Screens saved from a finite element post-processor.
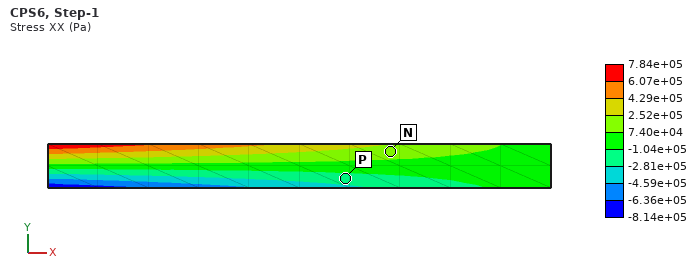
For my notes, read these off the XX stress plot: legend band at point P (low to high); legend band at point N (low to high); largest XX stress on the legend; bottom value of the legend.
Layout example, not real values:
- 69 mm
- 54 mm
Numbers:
- -2.81e+05 to -1.04e+05 Pa
- 7.40e+04 to 2.52e+05 Pa
- 7.84e+05 Pa
- -8.14e+05 Pa
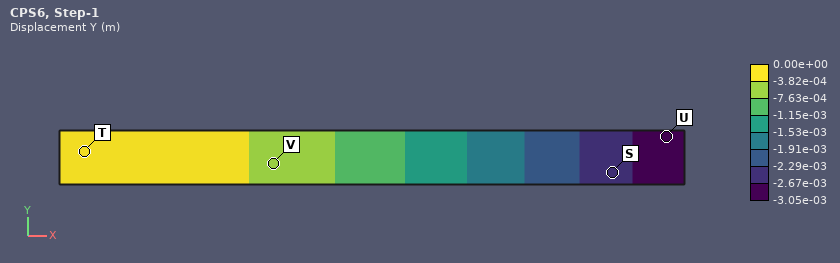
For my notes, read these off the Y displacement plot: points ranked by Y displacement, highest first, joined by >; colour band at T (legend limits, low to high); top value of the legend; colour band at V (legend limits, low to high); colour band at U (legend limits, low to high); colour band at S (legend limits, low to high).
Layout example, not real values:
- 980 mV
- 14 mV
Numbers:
- T > V > S > U
- -3.82e-04 to 0.00e+00 m
- 0.00e+00 m
- -7.63e-04 to -3.82e-04 m
- -3.05e-03 to -2.67e-03 m
- -2.67e-03 to -2.29e-03 m
